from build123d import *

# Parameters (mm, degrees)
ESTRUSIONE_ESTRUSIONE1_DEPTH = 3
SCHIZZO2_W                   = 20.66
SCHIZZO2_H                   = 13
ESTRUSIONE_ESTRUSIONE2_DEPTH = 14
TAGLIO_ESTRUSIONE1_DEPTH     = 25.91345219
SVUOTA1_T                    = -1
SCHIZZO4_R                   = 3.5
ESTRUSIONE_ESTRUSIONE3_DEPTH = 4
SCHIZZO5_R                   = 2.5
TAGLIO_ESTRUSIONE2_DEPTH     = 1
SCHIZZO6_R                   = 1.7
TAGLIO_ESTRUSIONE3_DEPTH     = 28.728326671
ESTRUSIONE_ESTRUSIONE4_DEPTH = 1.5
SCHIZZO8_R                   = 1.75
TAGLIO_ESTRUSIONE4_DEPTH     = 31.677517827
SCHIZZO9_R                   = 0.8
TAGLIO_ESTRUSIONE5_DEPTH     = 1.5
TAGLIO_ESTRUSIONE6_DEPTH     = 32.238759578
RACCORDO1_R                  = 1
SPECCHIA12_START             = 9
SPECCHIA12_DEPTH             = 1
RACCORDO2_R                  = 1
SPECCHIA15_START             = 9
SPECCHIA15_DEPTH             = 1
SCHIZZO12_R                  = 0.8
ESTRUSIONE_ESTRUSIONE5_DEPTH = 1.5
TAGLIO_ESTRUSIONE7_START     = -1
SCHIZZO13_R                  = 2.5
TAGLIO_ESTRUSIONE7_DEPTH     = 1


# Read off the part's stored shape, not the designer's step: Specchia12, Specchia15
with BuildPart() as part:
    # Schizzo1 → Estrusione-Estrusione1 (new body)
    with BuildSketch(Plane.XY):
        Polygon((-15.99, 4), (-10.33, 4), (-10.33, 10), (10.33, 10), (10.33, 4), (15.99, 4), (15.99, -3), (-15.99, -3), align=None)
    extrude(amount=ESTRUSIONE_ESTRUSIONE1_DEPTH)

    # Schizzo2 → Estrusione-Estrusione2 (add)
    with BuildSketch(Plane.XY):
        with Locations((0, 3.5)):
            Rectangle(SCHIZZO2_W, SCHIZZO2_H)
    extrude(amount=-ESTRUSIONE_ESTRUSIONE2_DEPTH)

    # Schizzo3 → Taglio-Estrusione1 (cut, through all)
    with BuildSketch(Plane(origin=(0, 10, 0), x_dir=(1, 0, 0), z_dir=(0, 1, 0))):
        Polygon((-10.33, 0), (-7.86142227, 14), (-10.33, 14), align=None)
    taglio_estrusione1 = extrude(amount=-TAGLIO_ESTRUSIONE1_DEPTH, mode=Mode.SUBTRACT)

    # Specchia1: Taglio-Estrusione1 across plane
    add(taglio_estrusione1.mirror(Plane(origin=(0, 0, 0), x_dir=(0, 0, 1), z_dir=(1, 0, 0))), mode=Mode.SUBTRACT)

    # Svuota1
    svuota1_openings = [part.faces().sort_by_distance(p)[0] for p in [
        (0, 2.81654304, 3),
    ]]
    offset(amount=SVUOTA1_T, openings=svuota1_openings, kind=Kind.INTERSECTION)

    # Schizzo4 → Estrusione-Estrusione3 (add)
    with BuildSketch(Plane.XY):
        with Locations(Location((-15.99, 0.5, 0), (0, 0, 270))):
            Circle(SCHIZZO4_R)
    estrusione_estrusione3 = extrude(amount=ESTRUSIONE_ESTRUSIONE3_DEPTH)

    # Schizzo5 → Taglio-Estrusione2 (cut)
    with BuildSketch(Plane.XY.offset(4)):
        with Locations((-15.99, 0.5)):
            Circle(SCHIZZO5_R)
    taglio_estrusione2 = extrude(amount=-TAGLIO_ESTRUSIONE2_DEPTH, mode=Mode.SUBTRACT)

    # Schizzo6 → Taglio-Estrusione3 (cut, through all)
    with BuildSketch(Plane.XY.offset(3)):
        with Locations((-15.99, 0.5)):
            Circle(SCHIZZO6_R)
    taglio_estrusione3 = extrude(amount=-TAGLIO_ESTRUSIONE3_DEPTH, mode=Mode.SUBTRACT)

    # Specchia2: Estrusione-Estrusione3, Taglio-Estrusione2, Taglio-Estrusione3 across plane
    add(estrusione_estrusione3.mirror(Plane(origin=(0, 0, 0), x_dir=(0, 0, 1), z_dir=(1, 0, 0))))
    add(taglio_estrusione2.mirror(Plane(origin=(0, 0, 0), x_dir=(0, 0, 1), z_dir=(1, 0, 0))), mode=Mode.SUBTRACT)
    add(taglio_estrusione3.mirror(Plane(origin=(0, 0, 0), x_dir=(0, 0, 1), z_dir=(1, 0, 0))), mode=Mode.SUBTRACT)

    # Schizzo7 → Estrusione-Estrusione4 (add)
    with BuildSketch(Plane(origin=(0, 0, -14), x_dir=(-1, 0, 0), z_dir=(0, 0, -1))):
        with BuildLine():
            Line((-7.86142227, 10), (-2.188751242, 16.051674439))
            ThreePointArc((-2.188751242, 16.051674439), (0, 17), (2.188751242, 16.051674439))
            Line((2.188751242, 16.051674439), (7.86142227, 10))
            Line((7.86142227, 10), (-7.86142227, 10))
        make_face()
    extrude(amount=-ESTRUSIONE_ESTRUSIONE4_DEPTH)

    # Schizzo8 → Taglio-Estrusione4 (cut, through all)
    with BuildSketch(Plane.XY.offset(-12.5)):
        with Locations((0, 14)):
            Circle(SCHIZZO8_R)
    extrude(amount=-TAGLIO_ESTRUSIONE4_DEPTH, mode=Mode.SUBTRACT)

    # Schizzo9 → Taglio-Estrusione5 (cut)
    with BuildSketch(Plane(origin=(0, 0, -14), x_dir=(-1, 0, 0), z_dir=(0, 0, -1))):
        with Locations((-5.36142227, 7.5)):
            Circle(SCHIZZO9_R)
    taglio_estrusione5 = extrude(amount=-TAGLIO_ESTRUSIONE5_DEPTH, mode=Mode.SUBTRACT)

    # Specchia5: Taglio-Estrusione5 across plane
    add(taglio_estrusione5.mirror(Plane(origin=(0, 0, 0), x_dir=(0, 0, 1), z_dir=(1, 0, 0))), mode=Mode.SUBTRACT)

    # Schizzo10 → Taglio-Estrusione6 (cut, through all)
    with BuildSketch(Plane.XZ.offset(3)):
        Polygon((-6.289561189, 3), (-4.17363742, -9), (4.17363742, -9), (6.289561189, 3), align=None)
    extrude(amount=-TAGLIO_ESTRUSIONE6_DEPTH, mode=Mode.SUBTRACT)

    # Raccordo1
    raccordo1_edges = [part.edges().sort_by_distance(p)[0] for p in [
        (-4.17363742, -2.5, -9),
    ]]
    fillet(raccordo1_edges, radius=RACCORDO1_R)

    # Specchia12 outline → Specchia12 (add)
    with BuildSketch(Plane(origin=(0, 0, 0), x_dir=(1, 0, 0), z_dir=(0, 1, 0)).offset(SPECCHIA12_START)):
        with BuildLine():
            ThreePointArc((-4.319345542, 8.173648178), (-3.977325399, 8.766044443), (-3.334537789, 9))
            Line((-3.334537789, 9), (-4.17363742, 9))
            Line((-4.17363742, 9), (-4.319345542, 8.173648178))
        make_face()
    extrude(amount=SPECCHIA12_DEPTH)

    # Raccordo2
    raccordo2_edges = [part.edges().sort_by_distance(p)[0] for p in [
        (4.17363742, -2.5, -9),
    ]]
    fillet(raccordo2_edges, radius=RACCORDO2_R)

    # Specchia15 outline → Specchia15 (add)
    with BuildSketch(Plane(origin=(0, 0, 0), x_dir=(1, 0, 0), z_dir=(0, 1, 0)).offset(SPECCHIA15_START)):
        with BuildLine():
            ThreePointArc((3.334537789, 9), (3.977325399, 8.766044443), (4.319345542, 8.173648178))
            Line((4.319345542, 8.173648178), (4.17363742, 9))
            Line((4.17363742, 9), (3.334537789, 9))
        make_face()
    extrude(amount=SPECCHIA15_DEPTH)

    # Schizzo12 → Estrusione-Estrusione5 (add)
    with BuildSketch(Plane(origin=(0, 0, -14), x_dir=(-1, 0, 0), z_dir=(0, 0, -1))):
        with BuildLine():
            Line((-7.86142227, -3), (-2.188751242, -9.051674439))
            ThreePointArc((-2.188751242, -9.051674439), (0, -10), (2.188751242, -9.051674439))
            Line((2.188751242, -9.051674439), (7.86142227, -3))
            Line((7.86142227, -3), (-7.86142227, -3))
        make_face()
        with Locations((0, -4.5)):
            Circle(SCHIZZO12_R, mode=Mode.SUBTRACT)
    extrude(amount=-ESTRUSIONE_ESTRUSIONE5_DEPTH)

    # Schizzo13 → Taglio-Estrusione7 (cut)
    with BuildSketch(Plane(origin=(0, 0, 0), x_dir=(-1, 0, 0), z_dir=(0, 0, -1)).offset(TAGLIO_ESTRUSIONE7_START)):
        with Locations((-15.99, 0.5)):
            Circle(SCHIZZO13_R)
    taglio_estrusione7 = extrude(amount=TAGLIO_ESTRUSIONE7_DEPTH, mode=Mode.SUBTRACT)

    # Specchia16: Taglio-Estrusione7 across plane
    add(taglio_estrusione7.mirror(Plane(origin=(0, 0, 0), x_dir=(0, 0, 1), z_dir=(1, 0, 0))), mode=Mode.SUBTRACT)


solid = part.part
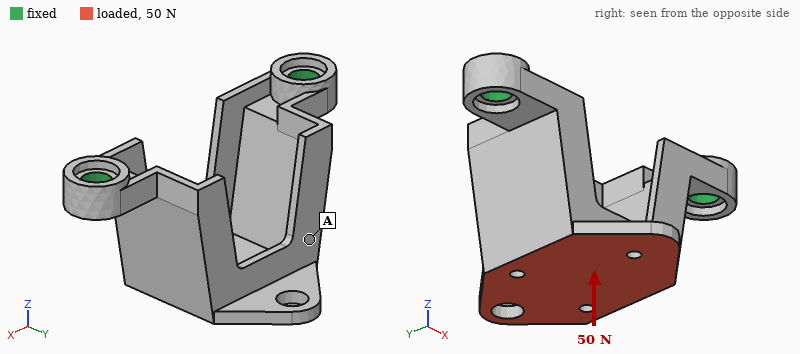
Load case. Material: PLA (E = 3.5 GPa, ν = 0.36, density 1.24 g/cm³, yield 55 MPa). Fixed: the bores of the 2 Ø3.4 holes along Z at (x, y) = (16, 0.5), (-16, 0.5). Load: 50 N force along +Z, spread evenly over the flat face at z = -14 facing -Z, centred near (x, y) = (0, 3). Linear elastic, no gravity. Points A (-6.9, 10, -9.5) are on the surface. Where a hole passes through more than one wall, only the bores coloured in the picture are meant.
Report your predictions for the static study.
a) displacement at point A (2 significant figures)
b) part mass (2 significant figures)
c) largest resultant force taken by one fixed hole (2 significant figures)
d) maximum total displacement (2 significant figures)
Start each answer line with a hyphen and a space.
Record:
- 0.25 mm
- 1.6 g
- 27 N
- 0.42 mm
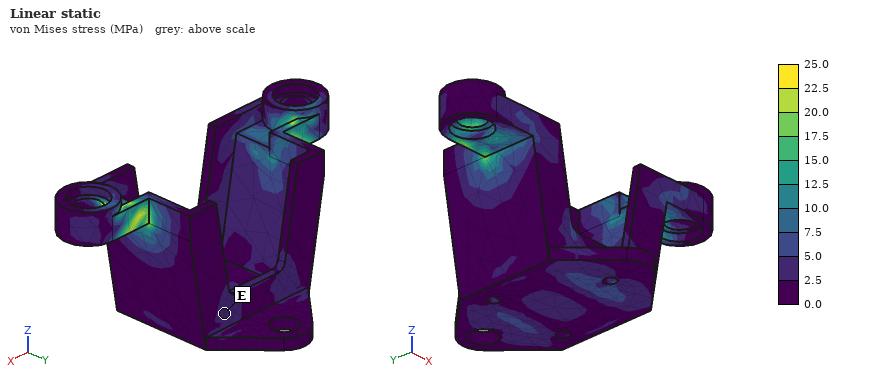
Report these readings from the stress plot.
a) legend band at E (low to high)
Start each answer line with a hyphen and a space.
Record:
- 2.5 to 5.0 MPa
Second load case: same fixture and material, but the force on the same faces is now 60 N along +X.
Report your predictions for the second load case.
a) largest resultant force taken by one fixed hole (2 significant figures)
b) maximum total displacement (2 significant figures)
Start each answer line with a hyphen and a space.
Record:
- 48 N
- 0.28 mm
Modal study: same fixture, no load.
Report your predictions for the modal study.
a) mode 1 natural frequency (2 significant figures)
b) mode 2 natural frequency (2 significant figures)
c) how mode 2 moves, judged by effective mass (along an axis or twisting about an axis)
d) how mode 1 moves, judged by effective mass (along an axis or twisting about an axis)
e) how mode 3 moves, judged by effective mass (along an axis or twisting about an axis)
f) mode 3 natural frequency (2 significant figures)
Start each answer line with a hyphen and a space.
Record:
- 1100 Hz
- 2200 Hz
- along X
- along Y
- along X
- 3700 Hz
